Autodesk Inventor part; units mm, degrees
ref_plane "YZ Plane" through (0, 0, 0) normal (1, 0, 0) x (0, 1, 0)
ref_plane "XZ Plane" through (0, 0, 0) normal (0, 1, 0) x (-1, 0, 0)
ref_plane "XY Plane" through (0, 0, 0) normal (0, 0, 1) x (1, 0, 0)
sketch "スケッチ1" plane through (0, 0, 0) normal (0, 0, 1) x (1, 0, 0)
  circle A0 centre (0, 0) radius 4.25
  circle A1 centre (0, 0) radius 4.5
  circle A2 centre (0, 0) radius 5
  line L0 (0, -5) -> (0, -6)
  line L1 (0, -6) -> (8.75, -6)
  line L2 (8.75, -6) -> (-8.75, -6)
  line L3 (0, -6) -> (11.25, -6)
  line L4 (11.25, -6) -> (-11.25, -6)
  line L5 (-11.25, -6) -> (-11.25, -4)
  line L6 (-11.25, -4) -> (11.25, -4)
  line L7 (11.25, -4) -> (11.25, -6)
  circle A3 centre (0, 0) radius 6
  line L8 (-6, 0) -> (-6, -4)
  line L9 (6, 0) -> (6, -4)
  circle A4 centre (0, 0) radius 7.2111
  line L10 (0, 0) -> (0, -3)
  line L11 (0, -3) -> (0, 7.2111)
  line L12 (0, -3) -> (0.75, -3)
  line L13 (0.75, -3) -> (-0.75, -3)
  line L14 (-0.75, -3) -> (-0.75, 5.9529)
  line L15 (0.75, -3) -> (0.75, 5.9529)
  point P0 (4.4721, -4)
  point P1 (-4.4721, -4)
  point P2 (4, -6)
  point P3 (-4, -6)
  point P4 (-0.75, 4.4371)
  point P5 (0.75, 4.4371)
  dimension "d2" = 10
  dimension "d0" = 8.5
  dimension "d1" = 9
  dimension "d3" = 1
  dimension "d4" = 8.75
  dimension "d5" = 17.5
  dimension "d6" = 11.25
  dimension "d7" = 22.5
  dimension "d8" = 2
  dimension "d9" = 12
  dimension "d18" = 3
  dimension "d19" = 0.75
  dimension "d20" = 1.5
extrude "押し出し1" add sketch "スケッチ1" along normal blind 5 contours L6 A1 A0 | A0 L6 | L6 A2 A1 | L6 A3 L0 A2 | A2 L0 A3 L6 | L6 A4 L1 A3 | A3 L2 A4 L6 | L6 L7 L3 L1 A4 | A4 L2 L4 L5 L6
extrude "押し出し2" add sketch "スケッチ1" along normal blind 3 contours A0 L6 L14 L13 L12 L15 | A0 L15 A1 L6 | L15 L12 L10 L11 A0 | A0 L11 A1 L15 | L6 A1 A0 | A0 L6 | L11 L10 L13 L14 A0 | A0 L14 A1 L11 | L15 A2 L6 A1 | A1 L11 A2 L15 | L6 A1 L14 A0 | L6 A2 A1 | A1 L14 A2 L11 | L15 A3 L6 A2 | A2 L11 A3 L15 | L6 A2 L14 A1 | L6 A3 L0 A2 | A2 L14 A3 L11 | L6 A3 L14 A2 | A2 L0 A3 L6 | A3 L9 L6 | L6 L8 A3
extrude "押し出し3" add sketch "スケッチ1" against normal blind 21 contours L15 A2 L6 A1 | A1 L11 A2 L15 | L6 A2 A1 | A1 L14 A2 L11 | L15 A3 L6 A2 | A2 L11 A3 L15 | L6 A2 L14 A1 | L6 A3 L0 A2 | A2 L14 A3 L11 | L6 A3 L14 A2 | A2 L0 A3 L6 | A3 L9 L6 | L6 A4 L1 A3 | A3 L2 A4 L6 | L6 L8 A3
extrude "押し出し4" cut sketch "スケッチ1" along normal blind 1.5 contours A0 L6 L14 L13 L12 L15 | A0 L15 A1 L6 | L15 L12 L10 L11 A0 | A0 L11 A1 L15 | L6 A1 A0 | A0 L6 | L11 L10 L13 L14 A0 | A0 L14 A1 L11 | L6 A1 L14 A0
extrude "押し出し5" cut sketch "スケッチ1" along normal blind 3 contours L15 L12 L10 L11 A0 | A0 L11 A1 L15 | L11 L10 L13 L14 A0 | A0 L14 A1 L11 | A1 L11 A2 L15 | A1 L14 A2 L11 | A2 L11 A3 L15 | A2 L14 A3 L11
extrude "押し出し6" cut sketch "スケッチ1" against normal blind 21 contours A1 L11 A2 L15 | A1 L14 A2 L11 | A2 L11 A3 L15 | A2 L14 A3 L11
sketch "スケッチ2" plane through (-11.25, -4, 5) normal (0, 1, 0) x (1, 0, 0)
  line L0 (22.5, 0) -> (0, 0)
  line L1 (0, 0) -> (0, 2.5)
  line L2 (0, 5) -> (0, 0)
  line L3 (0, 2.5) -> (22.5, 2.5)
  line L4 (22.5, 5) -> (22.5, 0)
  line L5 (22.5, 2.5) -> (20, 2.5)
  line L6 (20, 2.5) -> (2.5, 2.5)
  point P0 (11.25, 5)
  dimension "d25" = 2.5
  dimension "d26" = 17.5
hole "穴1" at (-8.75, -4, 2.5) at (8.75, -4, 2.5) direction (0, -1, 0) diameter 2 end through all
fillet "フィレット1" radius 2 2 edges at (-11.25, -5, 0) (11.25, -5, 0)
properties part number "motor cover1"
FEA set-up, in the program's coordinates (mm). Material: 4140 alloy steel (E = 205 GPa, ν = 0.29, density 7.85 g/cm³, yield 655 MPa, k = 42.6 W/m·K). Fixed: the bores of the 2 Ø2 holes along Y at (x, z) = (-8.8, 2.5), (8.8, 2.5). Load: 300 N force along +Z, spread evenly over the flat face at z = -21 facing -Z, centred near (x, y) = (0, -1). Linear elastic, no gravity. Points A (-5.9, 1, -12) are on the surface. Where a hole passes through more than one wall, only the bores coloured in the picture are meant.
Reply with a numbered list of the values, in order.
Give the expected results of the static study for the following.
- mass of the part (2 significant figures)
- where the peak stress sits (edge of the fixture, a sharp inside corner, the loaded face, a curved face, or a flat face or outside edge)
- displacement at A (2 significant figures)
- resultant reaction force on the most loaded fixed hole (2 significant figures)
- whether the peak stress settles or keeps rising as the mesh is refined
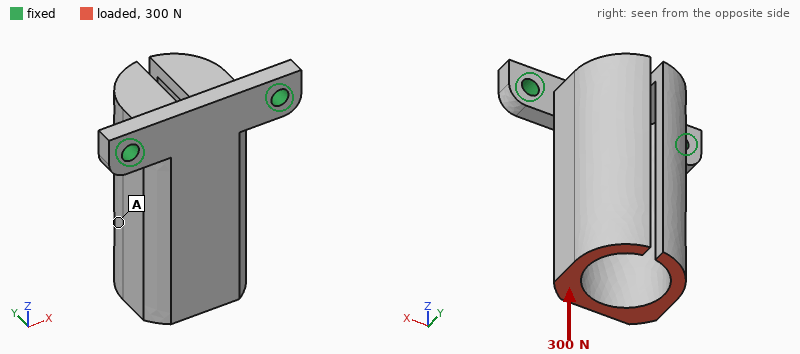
1. 13 g
2. edge of the fixture
3. 38 µm
4. 150 N
5. keeps rising
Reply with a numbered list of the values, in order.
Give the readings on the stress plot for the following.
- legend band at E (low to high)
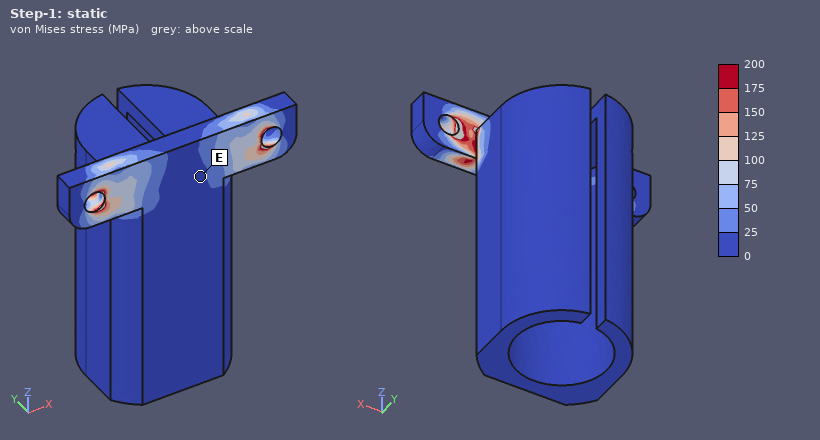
1. 0 to 25 MPa
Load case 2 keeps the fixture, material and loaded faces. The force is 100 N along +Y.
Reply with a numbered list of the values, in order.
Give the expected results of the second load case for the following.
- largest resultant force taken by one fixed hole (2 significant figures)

1. 79 N
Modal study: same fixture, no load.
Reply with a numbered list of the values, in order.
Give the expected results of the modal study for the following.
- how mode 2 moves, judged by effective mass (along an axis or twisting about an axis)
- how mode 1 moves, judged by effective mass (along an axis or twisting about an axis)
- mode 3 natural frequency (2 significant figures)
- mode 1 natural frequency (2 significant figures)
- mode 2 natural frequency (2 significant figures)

1. along X
2. along Y
3. 9700 Hz
4. 2300 Hz
5. 6000 Hz
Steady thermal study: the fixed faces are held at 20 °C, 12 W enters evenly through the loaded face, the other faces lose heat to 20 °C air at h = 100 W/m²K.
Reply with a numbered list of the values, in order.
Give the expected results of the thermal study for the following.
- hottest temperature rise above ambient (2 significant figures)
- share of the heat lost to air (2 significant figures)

1. 88 K
2. 68 %
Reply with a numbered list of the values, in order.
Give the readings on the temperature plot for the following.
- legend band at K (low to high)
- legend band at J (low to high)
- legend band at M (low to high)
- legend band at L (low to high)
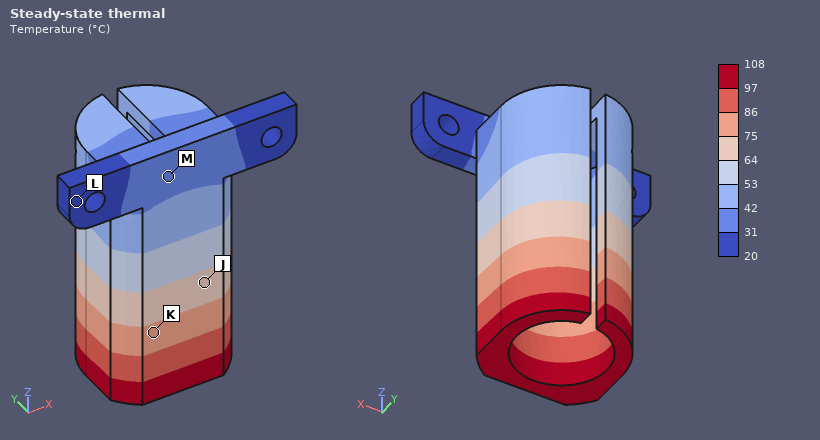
1. 75 to 86 °C
2. 64 to 75 °C
3. 31 to 42 °C
4. 20 to 31 °C
